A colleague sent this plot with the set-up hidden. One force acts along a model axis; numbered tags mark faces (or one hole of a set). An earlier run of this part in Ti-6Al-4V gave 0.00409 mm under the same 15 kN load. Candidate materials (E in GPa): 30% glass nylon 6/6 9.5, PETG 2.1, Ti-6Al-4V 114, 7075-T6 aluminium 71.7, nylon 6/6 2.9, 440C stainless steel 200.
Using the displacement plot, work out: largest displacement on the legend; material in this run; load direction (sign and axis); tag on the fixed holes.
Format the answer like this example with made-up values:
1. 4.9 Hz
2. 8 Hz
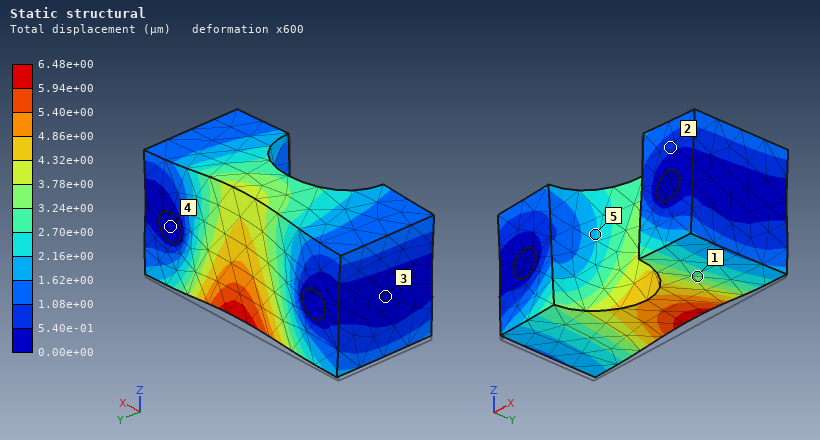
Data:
1. 6.48e+00 µm
2. 7075-T6 aluminium
3. +Z
4. 4
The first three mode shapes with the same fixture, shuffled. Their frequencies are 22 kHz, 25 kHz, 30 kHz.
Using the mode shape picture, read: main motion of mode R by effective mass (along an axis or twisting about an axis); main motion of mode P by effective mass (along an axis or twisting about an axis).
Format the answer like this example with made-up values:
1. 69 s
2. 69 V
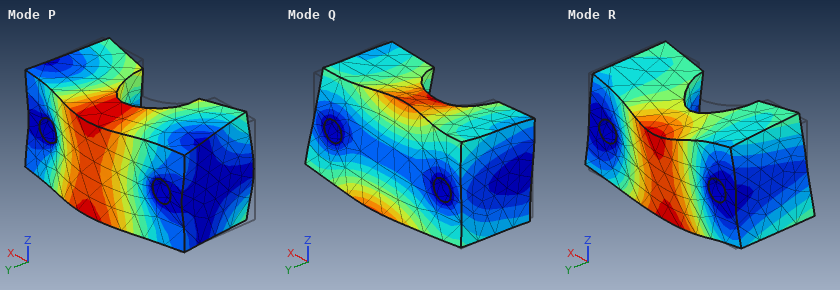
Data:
1. along Z
2. along Y
